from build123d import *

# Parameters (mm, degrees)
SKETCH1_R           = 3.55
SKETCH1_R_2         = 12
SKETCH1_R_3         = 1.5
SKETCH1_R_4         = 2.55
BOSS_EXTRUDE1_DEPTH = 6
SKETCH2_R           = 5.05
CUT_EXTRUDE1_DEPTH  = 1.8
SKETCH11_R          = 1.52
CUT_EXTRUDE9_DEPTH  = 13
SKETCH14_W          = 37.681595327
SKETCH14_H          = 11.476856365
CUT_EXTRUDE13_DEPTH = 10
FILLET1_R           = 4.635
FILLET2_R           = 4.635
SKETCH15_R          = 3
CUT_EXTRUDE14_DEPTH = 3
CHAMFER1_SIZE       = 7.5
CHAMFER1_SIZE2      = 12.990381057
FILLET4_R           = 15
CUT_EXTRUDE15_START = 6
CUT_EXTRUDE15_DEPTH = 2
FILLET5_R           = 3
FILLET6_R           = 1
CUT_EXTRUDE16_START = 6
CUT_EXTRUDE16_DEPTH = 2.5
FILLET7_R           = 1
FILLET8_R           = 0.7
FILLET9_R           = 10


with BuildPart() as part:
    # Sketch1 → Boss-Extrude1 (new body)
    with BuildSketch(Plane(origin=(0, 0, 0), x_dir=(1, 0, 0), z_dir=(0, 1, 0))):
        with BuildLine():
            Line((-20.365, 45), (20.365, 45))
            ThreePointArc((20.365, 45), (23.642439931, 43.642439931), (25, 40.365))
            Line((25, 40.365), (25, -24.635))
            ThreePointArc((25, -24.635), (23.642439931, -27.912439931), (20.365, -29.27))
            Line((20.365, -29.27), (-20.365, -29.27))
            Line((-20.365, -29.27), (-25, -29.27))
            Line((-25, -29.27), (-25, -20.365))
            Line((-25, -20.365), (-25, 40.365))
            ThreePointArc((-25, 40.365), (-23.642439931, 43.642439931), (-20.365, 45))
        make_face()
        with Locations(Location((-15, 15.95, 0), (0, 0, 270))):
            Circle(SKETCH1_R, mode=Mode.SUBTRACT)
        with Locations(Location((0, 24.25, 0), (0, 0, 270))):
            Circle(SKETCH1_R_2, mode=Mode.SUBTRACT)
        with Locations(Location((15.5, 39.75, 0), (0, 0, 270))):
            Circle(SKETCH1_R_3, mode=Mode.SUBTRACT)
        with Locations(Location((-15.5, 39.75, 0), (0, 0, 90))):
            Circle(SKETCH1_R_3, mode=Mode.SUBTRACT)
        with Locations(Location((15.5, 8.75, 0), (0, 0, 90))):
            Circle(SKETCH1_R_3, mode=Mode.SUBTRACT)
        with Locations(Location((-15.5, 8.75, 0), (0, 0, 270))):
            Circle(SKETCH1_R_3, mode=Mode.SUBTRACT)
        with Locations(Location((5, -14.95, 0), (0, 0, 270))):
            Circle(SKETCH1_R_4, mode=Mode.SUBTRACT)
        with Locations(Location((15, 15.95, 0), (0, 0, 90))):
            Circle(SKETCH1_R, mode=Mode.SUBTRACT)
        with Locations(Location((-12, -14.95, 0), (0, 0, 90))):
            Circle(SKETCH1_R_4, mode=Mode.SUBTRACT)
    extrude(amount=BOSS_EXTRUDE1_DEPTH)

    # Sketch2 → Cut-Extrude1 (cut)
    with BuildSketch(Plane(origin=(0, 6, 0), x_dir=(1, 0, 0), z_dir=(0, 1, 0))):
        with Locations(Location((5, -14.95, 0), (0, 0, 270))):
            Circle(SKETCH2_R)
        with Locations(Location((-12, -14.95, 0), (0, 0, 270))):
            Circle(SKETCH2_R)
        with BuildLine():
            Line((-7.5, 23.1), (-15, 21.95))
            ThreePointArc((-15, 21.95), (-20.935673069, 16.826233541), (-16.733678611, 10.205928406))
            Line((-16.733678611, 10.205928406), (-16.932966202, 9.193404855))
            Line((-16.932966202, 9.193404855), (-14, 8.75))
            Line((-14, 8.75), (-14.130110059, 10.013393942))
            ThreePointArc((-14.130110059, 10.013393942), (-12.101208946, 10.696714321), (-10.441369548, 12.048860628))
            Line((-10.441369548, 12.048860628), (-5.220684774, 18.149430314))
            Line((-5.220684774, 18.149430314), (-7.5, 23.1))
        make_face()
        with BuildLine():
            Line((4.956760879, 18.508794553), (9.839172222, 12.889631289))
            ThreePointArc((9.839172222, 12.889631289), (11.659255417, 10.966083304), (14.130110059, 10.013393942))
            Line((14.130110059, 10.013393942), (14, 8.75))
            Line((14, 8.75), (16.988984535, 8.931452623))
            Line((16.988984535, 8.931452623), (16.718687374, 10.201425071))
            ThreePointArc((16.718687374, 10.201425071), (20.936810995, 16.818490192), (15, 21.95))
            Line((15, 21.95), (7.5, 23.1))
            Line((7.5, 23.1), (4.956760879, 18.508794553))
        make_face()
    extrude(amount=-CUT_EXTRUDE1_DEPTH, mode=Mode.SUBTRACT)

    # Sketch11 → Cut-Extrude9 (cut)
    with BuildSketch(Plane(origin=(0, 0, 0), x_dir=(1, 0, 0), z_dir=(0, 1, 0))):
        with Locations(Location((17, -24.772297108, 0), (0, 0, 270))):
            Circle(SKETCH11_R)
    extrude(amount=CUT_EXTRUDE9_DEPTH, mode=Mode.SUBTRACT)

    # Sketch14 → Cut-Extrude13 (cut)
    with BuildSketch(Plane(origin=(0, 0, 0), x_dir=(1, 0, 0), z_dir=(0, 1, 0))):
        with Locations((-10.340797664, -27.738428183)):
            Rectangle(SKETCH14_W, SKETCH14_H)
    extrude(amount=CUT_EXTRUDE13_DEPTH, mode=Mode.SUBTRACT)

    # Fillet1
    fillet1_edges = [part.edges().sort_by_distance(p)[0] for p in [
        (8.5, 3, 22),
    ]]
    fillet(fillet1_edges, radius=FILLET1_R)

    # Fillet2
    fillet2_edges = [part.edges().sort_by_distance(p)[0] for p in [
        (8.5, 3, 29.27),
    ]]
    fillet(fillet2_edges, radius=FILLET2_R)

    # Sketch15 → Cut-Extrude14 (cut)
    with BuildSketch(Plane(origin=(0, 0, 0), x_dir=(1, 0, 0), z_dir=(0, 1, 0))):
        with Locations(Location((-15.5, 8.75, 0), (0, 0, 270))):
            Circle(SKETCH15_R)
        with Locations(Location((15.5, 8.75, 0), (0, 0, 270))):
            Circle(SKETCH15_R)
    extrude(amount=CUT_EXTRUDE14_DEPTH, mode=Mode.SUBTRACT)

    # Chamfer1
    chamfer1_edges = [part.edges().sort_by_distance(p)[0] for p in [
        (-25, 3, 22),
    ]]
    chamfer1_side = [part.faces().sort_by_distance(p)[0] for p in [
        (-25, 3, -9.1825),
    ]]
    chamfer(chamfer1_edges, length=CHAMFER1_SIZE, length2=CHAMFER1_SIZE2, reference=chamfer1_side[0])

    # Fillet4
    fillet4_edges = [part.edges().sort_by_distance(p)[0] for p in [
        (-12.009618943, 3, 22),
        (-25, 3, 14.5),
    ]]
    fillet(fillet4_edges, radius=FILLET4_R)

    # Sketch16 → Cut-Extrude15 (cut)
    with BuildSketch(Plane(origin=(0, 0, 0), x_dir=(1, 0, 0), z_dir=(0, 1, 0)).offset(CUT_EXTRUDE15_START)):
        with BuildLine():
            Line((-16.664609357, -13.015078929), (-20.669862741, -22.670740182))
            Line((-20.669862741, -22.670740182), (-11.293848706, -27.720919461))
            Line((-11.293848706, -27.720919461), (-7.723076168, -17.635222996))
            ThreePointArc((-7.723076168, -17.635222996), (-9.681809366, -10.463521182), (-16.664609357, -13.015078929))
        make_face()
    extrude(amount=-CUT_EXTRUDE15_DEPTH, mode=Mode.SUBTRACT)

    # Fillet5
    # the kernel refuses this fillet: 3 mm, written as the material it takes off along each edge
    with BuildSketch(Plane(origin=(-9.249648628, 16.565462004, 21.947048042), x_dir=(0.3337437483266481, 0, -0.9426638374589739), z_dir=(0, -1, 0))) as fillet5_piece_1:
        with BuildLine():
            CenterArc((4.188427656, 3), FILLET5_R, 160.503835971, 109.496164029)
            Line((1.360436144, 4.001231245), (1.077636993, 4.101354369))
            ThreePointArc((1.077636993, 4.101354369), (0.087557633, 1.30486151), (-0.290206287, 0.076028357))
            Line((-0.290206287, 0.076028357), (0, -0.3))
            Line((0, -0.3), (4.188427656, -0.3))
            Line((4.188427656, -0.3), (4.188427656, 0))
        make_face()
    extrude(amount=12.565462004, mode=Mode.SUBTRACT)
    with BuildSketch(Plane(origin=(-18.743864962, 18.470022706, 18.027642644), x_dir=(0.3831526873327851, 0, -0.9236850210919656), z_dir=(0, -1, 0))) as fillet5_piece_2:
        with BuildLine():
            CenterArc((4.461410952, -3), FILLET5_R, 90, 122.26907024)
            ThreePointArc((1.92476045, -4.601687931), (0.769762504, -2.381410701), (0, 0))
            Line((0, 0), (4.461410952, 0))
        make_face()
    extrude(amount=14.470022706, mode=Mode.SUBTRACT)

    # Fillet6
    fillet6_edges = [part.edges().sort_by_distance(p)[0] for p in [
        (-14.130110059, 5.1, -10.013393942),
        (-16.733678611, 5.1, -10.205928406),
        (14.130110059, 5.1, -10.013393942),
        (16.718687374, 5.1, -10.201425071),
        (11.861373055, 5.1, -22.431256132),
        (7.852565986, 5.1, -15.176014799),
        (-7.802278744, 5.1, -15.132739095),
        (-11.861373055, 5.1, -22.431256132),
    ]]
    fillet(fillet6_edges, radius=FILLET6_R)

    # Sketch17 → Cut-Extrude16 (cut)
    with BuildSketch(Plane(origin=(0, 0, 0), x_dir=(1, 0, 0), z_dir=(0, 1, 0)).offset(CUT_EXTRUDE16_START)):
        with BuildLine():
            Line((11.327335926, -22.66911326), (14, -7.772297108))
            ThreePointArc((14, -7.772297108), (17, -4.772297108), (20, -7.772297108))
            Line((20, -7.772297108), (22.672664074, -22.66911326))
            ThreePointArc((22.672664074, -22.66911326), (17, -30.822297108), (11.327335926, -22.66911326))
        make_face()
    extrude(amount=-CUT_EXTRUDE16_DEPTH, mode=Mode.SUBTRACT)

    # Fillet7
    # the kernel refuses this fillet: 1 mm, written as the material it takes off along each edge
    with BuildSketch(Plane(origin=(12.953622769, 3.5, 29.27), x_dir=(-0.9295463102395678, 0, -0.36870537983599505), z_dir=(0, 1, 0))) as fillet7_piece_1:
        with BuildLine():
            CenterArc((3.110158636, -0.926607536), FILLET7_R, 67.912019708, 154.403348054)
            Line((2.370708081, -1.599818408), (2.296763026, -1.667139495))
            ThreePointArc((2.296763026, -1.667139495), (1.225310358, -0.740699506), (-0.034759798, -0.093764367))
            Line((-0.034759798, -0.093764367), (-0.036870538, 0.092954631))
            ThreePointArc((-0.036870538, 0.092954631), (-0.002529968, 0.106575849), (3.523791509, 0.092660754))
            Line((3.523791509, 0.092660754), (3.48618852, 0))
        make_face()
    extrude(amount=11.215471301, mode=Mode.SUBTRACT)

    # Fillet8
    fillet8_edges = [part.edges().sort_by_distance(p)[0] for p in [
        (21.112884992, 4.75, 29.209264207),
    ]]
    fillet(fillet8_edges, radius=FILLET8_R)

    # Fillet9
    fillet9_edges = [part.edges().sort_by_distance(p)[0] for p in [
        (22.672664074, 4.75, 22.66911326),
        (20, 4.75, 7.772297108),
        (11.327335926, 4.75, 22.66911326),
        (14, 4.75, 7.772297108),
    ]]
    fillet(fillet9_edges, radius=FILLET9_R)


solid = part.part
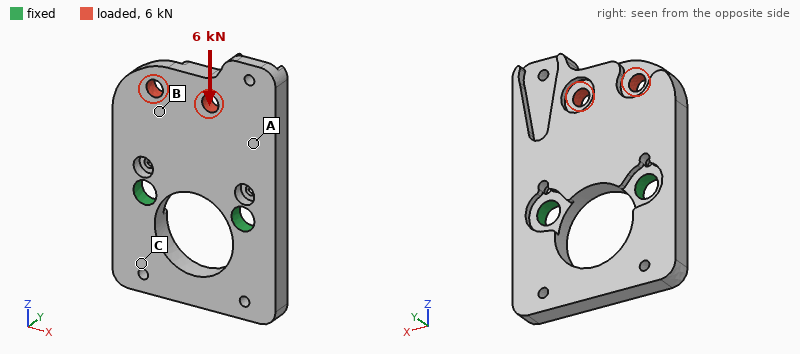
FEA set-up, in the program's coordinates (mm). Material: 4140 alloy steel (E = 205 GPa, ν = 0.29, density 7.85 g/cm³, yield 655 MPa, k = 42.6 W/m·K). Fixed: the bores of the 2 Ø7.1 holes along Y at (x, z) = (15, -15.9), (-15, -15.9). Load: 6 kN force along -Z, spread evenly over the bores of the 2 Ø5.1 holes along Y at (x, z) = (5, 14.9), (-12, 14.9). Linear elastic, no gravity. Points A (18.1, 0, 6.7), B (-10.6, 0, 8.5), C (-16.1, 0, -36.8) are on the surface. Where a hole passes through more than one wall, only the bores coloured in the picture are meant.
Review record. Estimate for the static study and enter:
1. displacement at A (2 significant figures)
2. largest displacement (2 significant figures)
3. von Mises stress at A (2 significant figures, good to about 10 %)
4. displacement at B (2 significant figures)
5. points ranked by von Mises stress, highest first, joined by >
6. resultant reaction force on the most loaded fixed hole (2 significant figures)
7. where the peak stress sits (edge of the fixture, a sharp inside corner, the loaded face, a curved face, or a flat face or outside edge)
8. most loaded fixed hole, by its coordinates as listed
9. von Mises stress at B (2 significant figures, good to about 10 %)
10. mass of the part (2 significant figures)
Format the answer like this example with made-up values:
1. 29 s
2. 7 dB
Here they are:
1. 9.5 µm
2. 30 µm
3. 25 MPa
4. 14 µm
5. B > A > C
6. 3.7 kN
7. a curved face
8. (-15, -15.9)
9. 55 MPa
10. 120 g
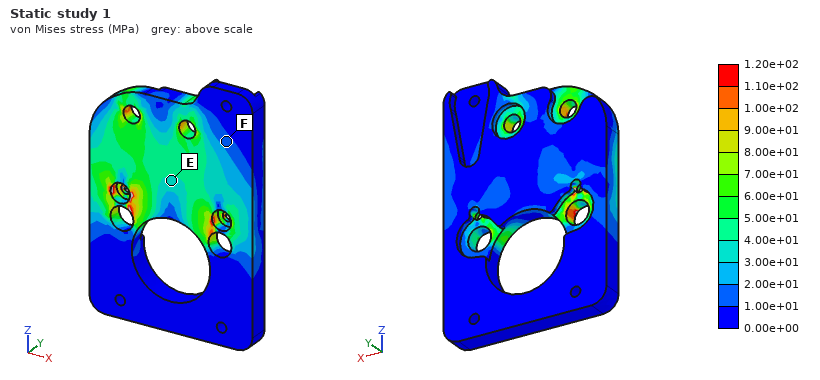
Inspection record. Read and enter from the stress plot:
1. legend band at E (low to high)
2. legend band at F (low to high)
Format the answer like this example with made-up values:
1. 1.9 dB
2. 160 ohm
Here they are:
1. 3.00e+01 to 4.00e+01 MPa
2. 1.00e+01 to 2.00e+01 MPa
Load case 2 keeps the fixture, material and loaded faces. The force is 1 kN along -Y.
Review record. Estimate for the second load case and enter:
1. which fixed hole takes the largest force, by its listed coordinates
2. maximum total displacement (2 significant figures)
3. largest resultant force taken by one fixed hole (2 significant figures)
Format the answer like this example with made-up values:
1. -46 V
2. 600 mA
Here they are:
1. (-15, -15.9)
2. 0.17 mm
3. 590 N
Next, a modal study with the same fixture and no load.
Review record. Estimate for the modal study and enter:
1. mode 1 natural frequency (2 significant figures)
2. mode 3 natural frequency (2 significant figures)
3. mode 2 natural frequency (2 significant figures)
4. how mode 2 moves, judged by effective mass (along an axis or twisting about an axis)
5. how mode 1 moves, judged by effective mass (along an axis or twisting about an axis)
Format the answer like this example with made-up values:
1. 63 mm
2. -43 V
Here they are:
1. 2500 Hz
2. 5900 Hz
3. 4100 Hz
4. along Y
5. along Y
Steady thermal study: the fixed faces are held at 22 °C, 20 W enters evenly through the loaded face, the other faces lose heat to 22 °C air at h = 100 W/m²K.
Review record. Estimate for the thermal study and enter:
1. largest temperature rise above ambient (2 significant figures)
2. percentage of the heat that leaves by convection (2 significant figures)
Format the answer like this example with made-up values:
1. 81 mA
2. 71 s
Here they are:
1. 52 K
2. 53 %
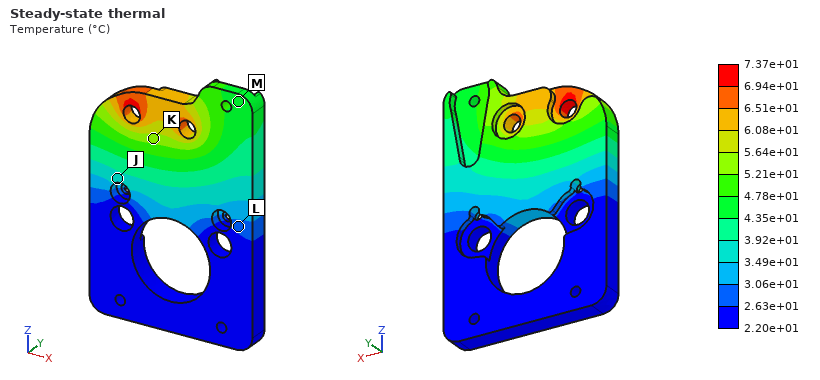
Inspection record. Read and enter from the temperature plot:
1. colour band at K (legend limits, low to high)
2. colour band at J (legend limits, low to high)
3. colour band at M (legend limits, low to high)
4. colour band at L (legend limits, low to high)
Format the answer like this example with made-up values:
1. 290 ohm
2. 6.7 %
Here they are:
1. 5.21e+01 to 5.64e+01 °C
2. 3.49e+01 to 3.92e+01 °C
3. 4.35e+01 to 4.78e+01 °C
4. 2.63e+01 to 3.06e+01 °C
